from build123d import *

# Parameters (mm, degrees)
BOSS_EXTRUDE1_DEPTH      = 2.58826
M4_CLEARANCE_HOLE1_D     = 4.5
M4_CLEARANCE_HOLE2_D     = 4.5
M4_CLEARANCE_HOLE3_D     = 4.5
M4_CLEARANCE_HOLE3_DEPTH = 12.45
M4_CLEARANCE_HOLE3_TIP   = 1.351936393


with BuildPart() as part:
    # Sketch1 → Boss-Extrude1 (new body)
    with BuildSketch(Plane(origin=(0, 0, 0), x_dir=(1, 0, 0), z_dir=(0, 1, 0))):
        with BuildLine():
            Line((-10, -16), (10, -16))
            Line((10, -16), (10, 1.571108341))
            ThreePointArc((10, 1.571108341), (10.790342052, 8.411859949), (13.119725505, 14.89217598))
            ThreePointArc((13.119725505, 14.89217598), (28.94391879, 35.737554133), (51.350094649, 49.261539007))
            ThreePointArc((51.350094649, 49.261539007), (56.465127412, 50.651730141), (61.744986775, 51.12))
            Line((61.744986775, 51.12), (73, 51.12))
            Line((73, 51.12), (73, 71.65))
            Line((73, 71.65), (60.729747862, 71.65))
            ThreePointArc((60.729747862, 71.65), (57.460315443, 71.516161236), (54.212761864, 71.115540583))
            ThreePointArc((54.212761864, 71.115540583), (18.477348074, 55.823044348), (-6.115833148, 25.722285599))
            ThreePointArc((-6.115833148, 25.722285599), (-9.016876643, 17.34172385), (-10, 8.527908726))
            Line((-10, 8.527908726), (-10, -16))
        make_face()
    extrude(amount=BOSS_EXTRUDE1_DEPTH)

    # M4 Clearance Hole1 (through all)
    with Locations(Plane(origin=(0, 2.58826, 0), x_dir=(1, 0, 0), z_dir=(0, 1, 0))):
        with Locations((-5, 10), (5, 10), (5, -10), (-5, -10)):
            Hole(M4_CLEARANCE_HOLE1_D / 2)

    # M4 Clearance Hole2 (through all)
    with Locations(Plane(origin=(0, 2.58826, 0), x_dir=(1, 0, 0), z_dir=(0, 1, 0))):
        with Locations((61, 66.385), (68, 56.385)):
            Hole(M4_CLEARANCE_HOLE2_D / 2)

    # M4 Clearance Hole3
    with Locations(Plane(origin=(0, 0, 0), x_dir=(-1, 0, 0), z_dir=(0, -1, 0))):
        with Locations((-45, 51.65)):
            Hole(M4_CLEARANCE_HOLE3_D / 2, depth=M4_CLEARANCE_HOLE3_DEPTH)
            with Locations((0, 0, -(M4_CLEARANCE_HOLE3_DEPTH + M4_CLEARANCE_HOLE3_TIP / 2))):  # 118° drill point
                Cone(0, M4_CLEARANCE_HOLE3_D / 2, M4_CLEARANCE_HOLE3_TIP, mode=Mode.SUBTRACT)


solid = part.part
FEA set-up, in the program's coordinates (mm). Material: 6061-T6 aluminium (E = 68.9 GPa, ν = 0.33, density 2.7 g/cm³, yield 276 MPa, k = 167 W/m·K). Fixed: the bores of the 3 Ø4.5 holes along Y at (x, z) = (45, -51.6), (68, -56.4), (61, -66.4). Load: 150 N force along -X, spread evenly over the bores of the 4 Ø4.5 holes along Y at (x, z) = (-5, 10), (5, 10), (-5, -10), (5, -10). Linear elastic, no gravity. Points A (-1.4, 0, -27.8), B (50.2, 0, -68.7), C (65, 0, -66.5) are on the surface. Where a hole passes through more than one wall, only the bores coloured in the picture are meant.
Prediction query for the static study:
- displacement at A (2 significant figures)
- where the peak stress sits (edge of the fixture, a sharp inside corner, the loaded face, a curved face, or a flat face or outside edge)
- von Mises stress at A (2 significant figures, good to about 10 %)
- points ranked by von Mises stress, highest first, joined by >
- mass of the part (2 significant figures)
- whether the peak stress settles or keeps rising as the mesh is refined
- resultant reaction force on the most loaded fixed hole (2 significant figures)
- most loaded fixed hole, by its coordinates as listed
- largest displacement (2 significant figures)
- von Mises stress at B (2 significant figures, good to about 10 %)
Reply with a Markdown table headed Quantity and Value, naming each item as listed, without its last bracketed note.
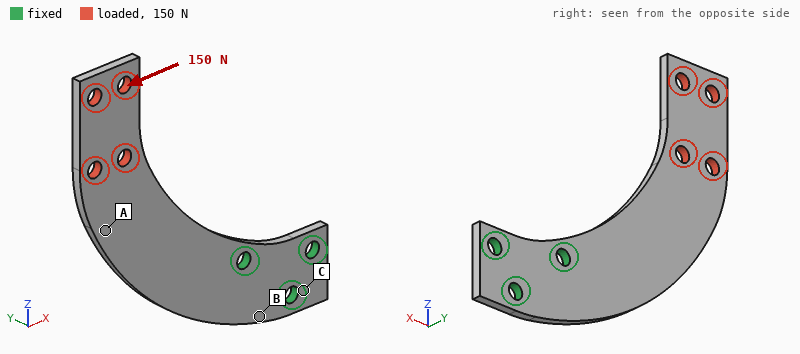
| Quantity | Value |
|---|---|
| displacement at A | 0.088 mm |
| where the peak stress sits | edge of the fixture |
| von Mises stress at A | 11 MPa |
| points ranked by von Mises stress, highest first, joined by > | B > A > C |
| mass of the part | 17 g |
| whether the peak stress settles or keeps rising as the mesh is refined | keeps rising |
| resultant reaction force on the most loaded fixed hole | 540 N |
| most loaded fixed hole, by its coordinates as listed | (45, -51.6) |
| largest displacement | 0.20 mm |
| von Mises stress at B | 18 MPa |
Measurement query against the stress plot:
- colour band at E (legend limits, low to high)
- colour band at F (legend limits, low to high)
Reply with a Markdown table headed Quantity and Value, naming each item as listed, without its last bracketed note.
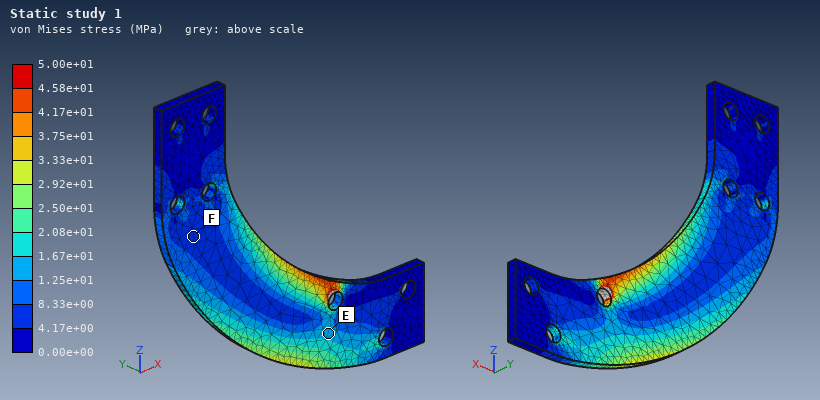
| Quantity | Value |
|---|---|
| colour band at E | 1.25e+01 to 1.67e+01 MPa |
| colour band at F | 4.17e+00 to 8.33e+00 MPa |
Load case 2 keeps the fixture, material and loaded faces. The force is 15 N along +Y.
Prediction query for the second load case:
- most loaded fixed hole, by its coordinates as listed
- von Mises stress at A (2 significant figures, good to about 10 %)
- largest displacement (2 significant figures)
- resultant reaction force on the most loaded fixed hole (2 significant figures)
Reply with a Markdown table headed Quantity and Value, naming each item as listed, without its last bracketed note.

| Quantity | Value |
|---|---|
| most loaded fixed hole, by its coordinates as listed | (45, -51.6) |
| von Mises stress at A | 13 MPa |
| largest displacement | 1.1 mm |
| resultant reaction force on the most loaded fixed hole | 26 N |
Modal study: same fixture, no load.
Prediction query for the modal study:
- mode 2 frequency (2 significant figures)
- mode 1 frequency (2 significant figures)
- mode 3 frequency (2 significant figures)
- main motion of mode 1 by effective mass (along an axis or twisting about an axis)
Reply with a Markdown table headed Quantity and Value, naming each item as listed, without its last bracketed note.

| Quantity | Value |
|---|---|
| mode 2 frequency | 1200 Hz |
| mode 1 frequency | 300 Hz |
| mode 3 frequency | 2000 Hz |
| main motion of mode 1 by effective mass | along Y |
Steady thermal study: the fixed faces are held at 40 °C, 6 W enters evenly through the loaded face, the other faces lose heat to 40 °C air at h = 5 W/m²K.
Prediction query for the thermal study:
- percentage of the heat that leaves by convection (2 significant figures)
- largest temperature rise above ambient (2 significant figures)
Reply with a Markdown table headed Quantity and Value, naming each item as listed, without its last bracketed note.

| Quantity | Value |
|---|---|
| percentage of the heat that leaves by convection | 9.6 % |
| largest temperature rise above ambient | 48 K |
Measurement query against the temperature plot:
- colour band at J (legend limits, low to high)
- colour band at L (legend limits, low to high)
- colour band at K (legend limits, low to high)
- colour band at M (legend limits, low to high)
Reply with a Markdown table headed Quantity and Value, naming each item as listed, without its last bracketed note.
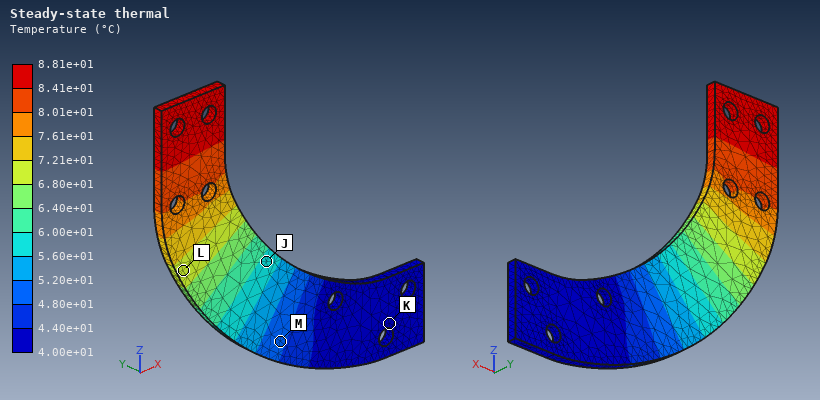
| Quantity | Value |
|---|---|
| colour band at J | 5.60e+01 to 6.00e+01 °C |
| colour band at L | 6.80e+01 to 7.21e+01 °C |
| colour band at K | 4.00e+01 to 4.40e+01 °C |
| colour band at M | 4.80e+01 to 5.20e+01 °C |
